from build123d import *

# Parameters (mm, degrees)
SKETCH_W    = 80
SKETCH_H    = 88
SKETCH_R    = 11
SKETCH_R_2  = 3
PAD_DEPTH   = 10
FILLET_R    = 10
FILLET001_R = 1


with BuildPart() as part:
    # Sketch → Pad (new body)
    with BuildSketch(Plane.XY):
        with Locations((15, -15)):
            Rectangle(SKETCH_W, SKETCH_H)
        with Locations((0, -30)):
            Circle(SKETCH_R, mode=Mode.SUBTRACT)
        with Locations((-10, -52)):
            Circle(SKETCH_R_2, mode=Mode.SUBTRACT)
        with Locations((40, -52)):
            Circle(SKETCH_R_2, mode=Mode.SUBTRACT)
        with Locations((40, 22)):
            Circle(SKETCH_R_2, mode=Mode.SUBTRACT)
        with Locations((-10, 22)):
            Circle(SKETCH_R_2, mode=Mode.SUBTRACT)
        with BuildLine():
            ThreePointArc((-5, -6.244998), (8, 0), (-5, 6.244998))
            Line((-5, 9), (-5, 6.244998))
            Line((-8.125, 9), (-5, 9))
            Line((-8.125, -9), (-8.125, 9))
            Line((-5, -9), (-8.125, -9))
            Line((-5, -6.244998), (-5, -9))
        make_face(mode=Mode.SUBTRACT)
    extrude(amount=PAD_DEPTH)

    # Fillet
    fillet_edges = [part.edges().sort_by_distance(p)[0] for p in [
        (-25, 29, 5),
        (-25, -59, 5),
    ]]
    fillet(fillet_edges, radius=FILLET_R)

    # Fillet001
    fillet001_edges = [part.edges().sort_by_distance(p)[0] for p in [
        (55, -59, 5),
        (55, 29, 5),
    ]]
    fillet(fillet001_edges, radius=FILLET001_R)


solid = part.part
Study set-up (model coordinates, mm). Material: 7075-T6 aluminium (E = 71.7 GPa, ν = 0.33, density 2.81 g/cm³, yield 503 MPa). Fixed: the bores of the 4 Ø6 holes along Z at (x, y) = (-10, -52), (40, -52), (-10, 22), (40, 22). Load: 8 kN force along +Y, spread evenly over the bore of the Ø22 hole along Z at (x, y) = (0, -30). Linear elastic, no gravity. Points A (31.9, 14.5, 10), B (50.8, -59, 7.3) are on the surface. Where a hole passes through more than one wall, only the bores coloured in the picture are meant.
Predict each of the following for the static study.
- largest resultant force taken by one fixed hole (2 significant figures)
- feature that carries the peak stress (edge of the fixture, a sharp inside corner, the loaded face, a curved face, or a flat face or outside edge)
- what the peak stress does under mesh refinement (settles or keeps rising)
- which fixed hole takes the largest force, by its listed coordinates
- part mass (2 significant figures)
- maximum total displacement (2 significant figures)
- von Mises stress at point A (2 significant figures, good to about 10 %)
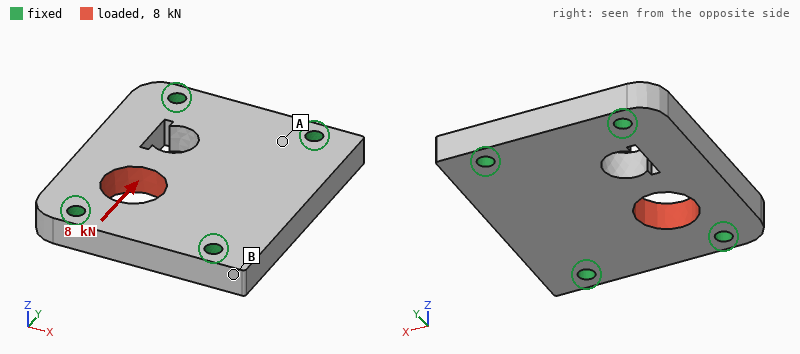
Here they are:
3.7 kN
edge of the fixture
keeps rising
(-10, -52)
180 g
8.8 µm
8.9 MPa
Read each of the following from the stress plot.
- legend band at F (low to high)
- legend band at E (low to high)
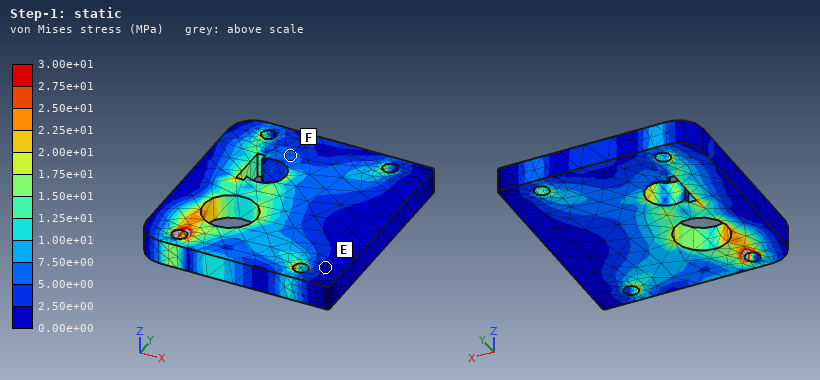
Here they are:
5.00e+00 to 7.50e+00 MPa
0.00e+00 to 2.50e+00 MPa
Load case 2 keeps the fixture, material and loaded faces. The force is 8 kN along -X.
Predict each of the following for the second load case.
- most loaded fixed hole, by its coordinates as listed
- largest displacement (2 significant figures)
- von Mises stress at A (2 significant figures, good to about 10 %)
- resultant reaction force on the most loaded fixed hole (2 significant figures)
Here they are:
(-10, -52)
14 µm
9.8 MPa
3.3 kN
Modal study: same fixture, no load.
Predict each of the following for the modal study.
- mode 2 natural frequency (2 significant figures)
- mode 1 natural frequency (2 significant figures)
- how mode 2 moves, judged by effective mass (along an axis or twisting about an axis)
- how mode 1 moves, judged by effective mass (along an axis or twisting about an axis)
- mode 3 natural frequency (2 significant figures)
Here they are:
8800 Hz
7300 Hz
twisting about Y
along Z
12 kHz
